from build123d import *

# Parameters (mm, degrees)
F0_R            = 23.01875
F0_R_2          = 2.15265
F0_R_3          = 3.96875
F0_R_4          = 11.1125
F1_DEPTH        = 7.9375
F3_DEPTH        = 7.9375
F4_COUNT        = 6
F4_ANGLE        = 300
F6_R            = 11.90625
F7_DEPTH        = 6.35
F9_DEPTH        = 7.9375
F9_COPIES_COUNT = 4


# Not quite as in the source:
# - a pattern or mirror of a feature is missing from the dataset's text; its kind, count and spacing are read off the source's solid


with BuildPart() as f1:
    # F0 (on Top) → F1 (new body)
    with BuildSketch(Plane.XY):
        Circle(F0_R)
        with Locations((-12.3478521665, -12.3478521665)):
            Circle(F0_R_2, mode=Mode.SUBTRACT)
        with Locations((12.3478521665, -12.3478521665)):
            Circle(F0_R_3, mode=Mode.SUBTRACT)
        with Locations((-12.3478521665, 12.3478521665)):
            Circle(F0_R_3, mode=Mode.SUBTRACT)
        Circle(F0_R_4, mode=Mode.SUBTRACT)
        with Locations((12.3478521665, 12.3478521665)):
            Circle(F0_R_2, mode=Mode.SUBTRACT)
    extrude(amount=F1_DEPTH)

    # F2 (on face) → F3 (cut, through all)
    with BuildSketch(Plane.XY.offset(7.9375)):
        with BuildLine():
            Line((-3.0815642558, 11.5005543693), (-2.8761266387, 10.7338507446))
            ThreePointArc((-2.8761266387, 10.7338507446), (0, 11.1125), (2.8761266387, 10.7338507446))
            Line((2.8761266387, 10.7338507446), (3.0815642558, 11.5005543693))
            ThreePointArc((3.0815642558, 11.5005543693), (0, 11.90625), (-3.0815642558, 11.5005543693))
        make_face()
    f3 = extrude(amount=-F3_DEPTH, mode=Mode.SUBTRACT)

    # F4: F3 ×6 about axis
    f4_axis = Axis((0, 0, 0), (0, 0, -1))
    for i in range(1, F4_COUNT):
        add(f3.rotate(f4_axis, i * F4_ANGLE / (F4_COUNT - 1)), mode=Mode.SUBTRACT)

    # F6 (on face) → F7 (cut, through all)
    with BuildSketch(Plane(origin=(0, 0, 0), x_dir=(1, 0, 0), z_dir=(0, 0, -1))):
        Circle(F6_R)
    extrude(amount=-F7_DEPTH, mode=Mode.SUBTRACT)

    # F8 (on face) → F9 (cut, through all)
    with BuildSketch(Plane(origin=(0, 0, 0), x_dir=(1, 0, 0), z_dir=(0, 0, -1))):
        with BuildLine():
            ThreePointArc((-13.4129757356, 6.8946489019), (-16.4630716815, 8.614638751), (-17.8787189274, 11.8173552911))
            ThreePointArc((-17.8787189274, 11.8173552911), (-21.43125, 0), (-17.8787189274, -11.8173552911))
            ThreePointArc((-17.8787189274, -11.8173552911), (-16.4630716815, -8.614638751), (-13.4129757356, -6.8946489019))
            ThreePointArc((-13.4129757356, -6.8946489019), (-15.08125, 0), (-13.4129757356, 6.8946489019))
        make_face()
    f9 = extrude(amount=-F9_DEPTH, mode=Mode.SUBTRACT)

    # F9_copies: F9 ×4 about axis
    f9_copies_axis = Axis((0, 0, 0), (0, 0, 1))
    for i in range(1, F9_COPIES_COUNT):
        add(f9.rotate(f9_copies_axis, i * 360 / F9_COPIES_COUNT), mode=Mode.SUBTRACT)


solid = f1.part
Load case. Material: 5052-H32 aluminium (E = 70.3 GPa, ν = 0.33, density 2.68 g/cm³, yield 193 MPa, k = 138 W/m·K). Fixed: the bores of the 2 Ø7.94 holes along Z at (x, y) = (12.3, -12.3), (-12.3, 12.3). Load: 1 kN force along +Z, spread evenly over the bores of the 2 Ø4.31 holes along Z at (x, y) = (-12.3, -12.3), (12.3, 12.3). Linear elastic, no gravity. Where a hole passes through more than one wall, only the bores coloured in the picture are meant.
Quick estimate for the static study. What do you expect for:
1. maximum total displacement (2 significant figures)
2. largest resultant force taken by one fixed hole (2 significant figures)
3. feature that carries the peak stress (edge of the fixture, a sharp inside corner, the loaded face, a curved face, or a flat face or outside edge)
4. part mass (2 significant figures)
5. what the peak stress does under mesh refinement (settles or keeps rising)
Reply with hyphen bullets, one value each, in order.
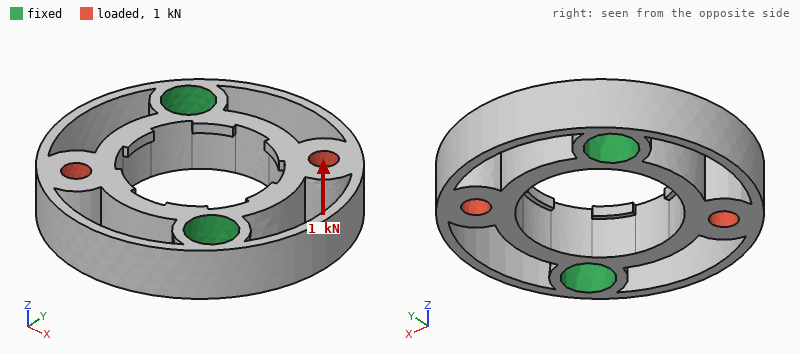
- 74 µm
- 500 N
- a sharp inside corner
- 14 g
- keeps rising
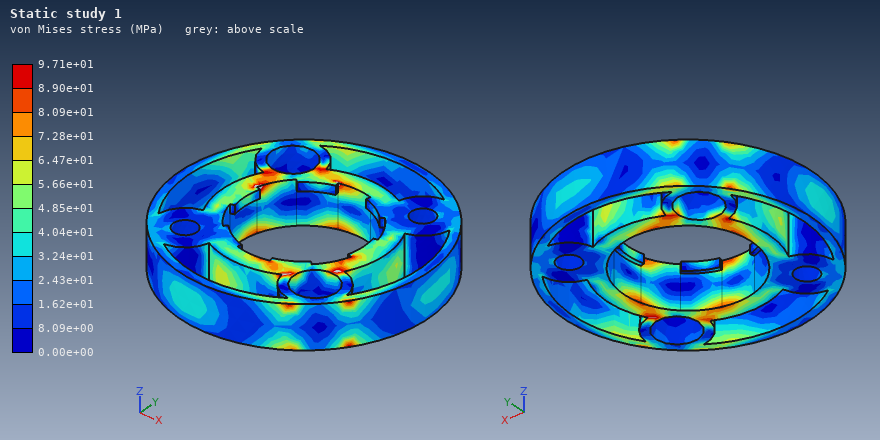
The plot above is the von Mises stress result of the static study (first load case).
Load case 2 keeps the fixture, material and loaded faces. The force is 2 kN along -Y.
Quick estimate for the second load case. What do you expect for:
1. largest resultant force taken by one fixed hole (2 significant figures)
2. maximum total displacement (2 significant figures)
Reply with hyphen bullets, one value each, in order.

- 1.0 kN
- 18 µm
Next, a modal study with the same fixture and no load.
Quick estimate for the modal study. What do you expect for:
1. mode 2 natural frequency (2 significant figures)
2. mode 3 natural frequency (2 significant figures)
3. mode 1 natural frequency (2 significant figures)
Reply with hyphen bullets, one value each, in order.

- 8500 Hz
- 16 kHz
- 8500 Hz
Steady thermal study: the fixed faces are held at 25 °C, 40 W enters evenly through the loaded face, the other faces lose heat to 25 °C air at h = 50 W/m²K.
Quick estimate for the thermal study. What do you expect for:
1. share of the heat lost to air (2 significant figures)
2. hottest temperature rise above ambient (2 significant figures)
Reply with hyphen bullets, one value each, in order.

- 10 %
- 38 K
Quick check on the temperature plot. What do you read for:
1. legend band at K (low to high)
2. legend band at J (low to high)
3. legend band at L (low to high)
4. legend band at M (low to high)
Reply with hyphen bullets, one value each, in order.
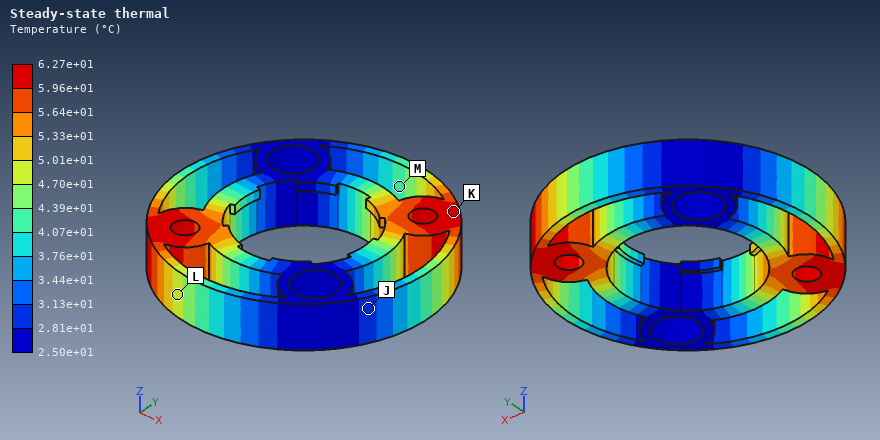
- 5.96e+01 to 6.27e+01 °C
- 2.81e+01 to 3.13e+01 °C
- 4.70e+01 to 5.01e+01 °C
- 4.07e+01 to 4.39e+01 °C
